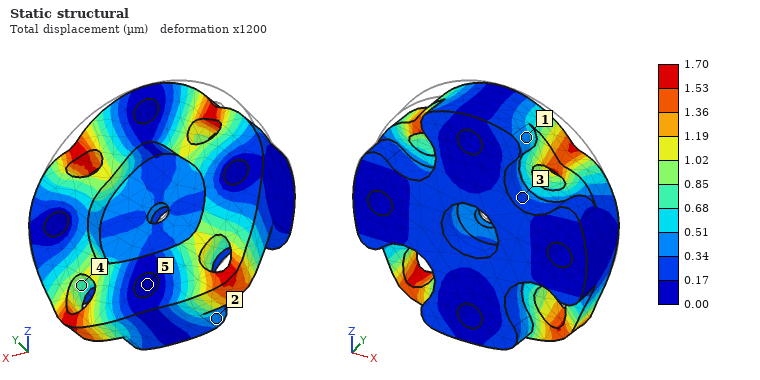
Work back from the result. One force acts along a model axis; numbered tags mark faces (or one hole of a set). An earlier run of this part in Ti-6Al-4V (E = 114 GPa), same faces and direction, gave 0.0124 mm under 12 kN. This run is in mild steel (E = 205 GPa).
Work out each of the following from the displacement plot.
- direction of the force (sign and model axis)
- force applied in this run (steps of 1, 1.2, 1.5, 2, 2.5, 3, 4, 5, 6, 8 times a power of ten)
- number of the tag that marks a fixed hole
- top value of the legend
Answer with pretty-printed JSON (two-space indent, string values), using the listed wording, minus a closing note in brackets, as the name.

{
  "direction of the force": "-Z",
  "force applied in this run": "3 kN",
  "number of the tag that marks a fixed hole": "5",
  "top value of the legend": "1.70 µm"
}
